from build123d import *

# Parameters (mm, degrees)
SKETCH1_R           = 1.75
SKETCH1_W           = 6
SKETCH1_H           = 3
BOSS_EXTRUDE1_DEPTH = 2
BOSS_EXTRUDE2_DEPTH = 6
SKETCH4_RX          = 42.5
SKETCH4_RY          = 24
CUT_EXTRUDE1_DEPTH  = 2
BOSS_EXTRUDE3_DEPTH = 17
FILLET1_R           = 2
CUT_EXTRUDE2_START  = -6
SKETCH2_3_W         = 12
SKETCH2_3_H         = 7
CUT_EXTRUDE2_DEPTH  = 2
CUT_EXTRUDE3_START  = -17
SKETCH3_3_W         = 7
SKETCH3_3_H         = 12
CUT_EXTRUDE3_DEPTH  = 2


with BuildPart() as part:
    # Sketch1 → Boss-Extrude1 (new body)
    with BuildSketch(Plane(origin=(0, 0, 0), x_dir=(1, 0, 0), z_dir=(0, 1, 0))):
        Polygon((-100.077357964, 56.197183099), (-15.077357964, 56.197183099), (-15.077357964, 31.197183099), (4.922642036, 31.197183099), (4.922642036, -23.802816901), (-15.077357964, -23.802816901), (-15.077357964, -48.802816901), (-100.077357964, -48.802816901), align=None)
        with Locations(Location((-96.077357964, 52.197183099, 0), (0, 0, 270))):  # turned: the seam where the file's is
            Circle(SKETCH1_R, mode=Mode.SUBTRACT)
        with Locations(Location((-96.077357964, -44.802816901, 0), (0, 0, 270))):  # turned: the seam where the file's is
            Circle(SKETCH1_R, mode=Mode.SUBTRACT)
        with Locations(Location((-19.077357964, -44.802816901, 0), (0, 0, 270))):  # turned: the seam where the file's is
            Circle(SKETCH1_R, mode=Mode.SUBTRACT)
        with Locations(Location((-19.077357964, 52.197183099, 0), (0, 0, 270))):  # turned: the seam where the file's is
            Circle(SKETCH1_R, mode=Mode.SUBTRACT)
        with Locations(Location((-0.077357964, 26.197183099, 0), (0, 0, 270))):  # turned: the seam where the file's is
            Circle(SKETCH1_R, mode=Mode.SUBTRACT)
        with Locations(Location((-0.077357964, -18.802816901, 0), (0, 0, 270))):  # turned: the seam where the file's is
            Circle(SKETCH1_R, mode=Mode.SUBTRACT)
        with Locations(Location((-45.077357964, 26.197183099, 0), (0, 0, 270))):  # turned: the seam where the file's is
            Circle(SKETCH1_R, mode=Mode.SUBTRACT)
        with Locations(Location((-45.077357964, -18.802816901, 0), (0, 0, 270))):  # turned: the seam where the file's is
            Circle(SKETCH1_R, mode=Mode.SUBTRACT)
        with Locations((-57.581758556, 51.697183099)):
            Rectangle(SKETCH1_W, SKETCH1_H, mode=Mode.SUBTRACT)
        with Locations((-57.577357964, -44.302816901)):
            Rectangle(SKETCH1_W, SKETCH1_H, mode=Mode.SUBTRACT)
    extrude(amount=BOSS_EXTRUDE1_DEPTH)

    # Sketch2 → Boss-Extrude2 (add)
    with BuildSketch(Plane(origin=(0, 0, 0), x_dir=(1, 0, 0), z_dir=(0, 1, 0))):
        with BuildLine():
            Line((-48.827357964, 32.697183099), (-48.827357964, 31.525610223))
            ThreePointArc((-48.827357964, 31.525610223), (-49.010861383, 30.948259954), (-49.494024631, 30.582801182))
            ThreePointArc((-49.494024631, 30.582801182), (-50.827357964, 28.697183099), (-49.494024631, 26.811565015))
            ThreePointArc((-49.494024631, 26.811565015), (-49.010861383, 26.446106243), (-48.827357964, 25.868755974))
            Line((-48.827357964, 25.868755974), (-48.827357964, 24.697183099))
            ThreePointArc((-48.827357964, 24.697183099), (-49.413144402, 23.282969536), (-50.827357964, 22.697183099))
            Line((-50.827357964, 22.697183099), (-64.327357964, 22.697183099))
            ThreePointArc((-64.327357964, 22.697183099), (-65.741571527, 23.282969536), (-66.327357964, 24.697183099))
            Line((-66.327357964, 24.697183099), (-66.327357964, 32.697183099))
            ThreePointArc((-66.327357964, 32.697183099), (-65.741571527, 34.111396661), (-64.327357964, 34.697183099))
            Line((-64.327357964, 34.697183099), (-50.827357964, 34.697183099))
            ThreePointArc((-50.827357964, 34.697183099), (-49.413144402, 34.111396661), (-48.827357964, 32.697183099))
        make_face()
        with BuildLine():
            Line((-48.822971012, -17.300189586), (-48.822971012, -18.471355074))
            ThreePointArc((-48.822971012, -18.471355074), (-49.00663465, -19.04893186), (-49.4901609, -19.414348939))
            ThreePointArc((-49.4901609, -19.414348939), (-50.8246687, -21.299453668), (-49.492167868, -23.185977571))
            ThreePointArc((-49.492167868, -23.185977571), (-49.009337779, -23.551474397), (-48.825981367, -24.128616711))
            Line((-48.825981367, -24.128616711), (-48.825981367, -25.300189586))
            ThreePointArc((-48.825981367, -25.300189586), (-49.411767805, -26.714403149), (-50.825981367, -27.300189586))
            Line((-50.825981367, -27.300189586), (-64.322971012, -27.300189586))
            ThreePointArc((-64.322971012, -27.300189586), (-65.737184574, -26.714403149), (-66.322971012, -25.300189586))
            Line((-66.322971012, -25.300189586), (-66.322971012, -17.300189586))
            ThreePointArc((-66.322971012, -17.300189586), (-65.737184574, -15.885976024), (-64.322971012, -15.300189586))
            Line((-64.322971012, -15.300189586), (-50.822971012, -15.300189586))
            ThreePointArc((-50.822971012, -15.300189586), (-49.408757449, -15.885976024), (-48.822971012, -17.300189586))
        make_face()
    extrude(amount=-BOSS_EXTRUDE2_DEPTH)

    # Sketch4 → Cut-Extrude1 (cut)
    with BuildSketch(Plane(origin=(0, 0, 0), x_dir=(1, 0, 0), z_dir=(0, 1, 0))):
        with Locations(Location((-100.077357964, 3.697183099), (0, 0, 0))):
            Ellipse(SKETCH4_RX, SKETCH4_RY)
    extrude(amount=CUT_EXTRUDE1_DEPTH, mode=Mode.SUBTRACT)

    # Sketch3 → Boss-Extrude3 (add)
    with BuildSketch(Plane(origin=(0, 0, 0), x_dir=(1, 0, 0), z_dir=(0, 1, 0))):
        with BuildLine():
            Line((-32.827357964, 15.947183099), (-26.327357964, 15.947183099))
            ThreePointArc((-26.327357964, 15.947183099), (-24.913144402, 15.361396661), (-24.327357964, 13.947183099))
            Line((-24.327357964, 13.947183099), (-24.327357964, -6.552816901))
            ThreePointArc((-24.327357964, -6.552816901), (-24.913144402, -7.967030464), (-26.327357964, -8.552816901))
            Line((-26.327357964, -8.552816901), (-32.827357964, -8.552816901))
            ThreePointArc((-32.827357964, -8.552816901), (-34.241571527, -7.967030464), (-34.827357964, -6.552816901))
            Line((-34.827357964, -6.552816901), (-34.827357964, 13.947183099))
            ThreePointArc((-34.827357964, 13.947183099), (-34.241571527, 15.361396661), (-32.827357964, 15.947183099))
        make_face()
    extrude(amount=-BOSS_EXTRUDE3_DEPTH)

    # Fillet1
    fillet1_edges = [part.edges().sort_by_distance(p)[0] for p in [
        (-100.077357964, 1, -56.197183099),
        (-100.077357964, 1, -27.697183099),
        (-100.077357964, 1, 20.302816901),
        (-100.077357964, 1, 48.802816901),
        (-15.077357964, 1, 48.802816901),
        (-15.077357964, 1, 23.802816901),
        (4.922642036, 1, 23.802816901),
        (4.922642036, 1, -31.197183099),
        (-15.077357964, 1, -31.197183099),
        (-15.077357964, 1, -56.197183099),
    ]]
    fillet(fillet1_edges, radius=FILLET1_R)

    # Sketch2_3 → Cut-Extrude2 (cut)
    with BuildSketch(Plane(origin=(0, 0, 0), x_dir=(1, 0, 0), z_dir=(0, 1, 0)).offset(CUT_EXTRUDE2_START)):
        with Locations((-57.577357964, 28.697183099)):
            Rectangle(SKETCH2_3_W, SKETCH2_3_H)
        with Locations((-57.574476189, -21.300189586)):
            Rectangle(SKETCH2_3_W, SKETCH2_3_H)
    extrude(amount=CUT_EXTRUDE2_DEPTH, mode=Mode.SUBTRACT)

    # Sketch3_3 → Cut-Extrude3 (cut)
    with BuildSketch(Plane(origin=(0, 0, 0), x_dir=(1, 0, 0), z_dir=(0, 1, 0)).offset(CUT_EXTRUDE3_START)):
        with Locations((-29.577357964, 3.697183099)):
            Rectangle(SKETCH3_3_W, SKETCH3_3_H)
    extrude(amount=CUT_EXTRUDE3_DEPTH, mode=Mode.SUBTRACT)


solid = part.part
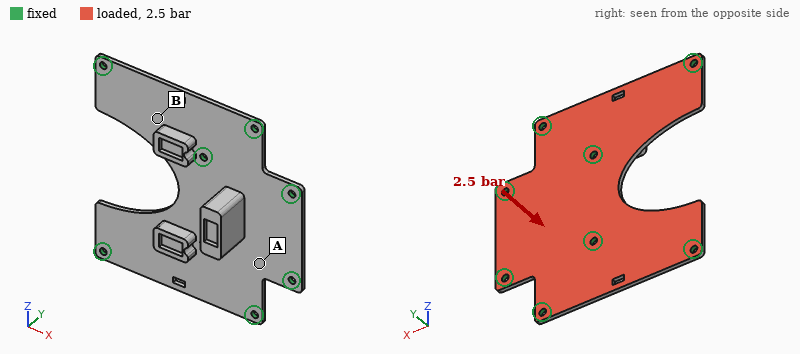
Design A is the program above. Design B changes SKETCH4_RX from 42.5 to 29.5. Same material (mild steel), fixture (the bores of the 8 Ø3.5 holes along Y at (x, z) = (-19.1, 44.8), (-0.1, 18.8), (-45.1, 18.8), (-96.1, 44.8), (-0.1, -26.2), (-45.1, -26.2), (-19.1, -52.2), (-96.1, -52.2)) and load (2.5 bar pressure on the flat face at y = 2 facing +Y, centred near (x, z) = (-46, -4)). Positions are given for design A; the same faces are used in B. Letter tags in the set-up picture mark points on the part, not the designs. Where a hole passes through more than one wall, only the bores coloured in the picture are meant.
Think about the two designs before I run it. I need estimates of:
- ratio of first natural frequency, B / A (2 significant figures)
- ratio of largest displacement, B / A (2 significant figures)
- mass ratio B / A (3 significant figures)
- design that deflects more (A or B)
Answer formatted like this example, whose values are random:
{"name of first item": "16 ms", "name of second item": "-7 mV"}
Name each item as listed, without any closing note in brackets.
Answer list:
{"ratio of first natural frequency, B / A": "0.91", "ratio of largest displacement, B / A": "1.3", "mass ratio B / A": "1.04", "design that deflects more": "B"}
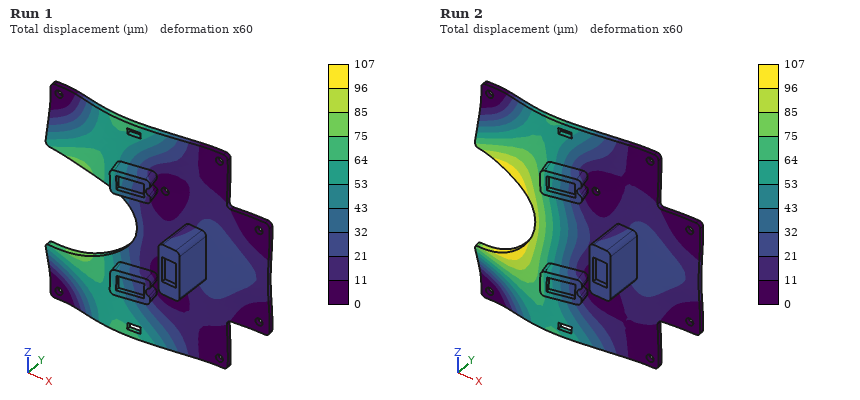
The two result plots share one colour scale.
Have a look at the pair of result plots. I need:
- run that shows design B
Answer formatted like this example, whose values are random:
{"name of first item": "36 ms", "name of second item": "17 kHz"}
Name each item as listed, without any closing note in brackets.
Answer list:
{"run that shows design B": "Run 2"}
